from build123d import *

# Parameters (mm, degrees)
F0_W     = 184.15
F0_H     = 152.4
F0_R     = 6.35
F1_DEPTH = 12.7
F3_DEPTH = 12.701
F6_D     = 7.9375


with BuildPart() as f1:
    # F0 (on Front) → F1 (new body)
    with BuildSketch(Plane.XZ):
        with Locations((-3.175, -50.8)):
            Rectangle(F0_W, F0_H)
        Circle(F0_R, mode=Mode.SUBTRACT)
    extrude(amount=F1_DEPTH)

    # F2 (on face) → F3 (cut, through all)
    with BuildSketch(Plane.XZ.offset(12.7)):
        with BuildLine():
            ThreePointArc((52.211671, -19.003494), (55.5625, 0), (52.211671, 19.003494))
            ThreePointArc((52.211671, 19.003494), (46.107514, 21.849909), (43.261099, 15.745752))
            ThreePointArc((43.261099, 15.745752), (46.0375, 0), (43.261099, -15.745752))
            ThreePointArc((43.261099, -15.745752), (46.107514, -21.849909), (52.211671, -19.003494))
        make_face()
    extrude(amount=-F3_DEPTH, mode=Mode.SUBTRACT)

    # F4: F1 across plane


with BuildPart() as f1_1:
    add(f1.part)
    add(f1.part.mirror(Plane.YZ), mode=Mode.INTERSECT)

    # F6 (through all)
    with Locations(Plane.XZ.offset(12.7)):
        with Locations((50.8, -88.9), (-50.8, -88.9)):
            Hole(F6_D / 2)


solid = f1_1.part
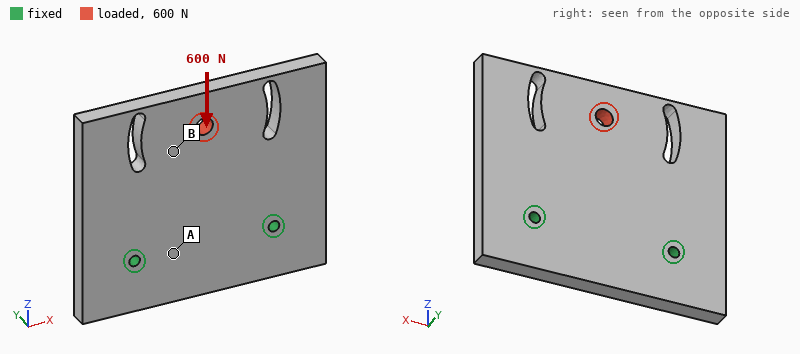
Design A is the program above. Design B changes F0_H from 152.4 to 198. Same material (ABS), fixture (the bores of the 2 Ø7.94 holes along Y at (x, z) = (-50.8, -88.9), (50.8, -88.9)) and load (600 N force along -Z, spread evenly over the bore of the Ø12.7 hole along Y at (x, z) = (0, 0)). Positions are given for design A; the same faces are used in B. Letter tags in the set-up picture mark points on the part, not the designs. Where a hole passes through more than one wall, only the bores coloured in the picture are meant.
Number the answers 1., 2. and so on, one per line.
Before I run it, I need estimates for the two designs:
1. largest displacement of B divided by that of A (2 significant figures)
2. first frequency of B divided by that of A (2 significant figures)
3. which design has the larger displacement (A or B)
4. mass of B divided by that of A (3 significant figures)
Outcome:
1. 0.86
2. 0.70
3. A
4. 1.31
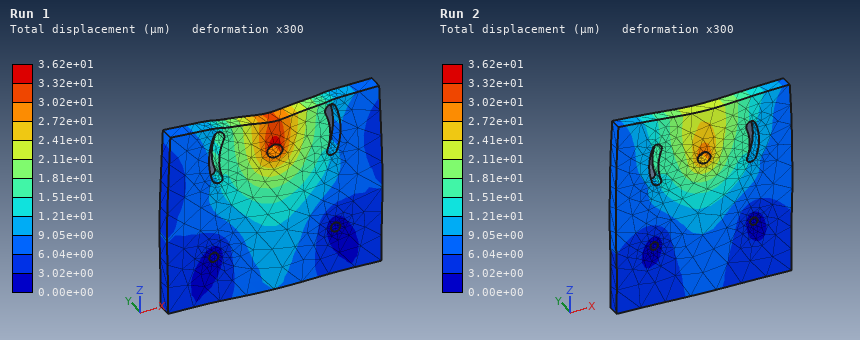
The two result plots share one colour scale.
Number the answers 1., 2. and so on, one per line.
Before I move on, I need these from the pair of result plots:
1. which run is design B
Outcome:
1. Run 2
